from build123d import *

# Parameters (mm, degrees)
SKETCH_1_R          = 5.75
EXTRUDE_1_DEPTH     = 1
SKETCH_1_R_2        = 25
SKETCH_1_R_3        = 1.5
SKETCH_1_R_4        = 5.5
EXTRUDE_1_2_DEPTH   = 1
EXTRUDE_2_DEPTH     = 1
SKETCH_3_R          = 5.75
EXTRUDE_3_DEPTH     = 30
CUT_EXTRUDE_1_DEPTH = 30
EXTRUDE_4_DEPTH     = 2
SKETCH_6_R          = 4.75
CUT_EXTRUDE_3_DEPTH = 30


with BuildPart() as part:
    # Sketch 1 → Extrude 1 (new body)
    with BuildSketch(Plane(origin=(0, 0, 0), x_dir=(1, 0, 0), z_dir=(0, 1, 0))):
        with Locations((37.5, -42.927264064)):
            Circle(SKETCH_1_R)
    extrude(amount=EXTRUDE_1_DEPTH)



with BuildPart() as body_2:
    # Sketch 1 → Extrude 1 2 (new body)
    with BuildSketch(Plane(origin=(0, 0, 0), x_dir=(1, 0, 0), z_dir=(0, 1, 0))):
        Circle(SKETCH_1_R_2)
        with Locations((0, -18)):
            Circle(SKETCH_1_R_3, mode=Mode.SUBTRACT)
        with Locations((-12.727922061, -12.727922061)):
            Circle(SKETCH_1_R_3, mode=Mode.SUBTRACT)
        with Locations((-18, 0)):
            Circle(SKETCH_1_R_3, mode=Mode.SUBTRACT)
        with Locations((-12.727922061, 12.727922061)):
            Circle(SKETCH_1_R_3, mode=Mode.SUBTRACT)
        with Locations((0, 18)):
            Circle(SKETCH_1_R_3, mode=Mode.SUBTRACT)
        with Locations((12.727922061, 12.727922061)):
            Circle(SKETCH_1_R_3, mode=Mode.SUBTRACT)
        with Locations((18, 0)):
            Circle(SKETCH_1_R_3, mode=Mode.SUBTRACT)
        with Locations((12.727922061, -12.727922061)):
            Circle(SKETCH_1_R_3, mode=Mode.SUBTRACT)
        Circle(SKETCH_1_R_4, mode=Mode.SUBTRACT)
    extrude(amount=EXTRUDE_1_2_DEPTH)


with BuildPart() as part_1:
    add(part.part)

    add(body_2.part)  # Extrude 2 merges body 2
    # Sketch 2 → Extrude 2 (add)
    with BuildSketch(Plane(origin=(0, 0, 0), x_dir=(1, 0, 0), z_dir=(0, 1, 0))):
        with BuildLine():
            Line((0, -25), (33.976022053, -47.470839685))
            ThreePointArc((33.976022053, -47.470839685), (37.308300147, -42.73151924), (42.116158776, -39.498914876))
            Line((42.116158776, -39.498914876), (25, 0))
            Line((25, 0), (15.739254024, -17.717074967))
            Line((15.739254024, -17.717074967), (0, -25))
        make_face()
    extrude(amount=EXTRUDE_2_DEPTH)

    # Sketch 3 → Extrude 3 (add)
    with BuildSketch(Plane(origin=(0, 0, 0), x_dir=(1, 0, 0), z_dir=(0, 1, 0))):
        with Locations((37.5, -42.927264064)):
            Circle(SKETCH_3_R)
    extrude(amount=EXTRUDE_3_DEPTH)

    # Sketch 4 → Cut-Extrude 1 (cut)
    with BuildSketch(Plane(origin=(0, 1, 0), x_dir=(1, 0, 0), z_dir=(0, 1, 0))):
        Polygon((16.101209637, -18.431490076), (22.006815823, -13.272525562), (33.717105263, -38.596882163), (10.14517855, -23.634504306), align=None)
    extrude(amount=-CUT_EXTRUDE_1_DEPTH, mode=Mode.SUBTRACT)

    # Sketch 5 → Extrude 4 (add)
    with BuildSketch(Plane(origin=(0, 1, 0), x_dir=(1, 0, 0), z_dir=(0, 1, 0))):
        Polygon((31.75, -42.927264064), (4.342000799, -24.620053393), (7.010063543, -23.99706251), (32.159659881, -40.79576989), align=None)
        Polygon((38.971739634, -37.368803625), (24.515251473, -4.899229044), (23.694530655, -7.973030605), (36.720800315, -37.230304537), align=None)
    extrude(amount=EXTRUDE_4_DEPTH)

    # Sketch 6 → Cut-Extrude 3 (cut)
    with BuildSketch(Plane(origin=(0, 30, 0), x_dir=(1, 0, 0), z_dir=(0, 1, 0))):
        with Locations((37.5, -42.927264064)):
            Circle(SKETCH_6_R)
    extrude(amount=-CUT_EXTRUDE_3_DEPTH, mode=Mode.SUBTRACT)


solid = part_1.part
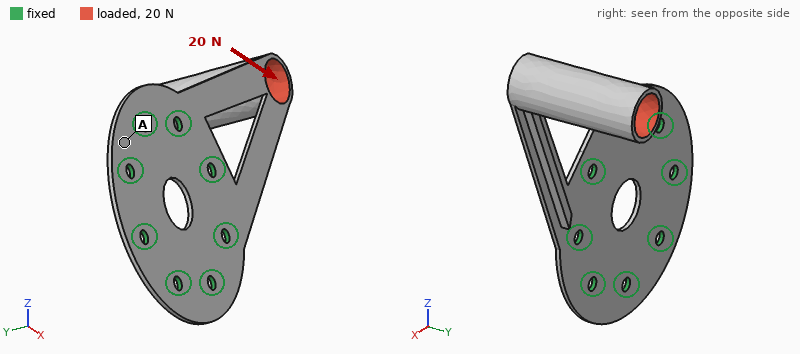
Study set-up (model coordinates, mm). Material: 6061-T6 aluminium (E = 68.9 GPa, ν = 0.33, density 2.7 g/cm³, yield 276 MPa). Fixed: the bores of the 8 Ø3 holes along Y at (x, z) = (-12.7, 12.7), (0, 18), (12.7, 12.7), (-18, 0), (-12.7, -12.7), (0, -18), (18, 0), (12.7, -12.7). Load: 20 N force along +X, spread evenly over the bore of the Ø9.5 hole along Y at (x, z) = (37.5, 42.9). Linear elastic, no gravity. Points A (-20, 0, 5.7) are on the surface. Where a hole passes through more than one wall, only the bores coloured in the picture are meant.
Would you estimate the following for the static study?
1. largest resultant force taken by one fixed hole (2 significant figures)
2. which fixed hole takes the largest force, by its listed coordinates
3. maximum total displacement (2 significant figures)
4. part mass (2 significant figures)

28 N
(0, 18)
0.73 mm
9.6 g
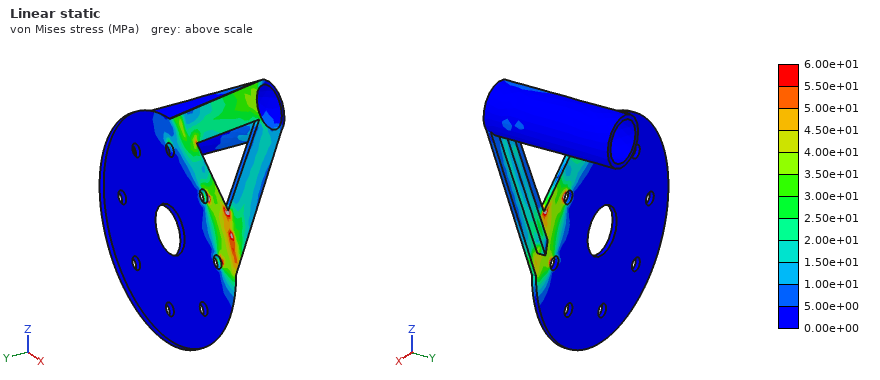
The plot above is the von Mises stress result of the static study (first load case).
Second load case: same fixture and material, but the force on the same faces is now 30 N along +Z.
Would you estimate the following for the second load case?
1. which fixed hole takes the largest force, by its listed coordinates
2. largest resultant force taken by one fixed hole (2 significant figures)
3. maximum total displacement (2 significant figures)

(18, 0)
39 N
1.1 mm
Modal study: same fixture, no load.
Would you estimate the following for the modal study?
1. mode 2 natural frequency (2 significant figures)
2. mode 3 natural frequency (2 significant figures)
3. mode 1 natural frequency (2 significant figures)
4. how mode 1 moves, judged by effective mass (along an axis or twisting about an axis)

730 Hz
1700 Hz
310 Hz
along Y
